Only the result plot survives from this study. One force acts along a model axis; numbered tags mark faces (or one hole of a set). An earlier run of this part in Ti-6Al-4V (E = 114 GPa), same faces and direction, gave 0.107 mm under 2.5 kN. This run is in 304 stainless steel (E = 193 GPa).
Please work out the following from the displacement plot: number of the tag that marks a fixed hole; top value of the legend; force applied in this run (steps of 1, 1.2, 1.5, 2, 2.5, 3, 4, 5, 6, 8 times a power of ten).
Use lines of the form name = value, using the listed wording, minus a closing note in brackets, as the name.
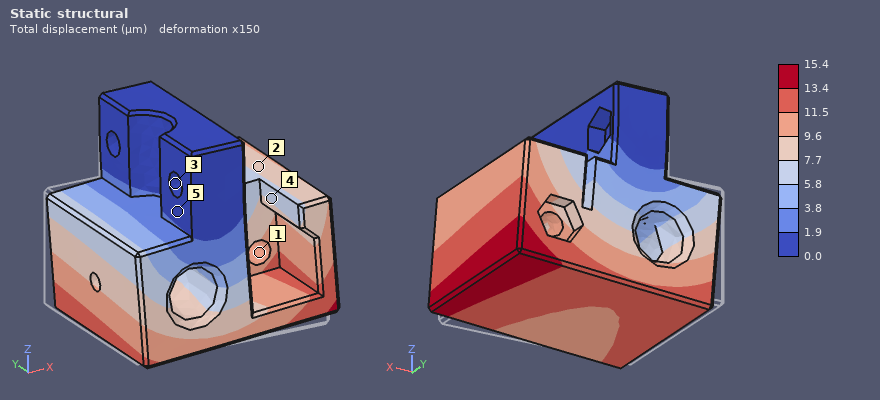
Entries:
number of the tag that marks a fixed hole = 3
top value of the legend = 15.4 µm
force applied in this run = 600 N
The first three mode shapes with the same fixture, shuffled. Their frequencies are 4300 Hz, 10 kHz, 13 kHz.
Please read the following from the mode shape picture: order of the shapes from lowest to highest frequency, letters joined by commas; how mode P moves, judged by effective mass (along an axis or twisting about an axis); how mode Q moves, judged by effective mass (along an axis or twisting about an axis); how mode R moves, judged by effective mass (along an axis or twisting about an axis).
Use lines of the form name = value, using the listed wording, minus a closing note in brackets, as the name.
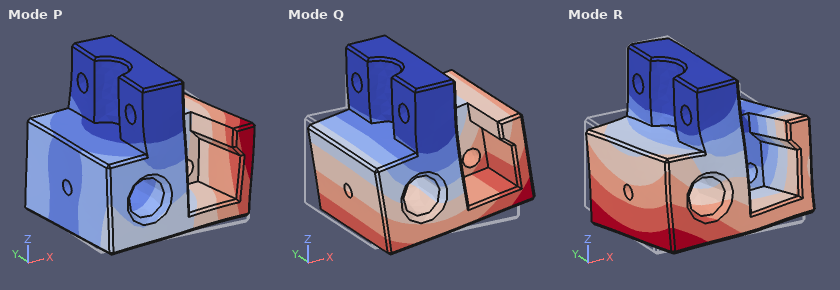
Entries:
order of the shapes from lowest to highest frequency, letters joined by commas = Q, P, R
how mode P moves, judged by effective mass = along Y
how mode Q moves, judged by effective mass = along X
how mode R moves, judged by effective mass = along Y
